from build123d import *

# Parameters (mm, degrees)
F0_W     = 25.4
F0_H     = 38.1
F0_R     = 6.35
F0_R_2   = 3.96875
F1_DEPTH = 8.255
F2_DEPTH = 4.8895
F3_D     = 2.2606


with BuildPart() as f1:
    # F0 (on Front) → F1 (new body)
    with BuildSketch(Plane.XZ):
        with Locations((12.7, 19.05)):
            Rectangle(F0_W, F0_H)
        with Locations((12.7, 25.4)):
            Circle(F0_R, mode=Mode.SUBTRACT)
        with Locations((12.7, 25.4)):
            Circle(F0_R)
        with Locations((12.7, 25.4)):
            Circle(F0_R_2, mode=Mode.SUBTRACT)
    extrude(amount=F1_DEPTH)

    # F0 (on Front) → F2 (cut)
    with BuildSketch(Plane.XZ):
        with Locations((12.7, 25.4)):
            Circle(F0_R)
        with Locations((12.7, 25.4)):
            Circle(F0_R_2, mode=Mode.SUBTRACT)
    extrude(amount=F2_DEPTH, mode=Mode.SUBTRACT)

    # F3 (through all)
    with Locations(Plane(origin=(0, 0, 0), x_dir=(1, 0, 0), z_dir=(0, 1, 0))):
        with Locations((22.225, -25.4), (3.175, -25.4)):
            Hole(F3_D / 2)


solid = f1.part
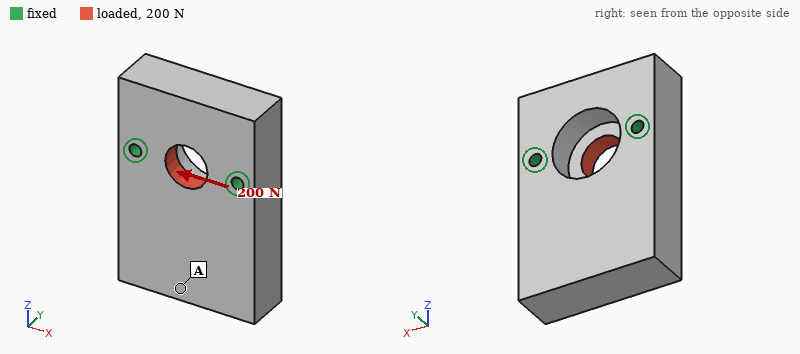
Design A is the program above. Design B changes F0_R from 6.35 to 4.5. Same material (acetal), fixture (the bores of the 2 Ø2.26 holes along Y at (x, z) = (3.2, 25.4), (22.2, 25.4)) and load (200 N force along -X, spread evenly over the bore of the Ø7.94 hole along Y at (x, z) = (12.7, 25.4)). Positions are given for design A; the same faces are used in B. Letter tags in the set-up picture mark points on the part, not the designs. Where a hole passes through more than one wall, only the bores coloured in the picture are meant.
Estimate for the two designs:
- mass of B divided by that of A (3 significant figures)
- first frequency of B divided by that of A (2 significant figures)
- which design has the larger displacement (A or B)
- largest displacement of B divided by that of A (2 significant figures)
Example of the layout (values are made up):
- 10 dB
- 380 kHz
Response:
- 1.04
- 1.0
- A
- 0.85
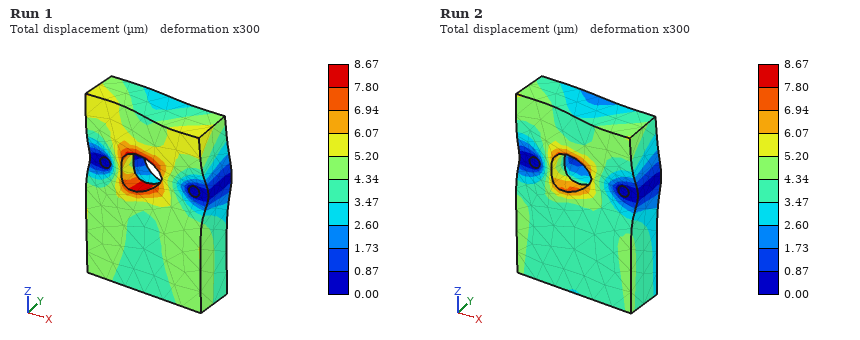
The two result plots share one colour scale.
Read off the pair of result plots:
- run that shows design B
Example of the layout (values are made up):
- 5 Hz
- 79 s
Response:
- Run 2
